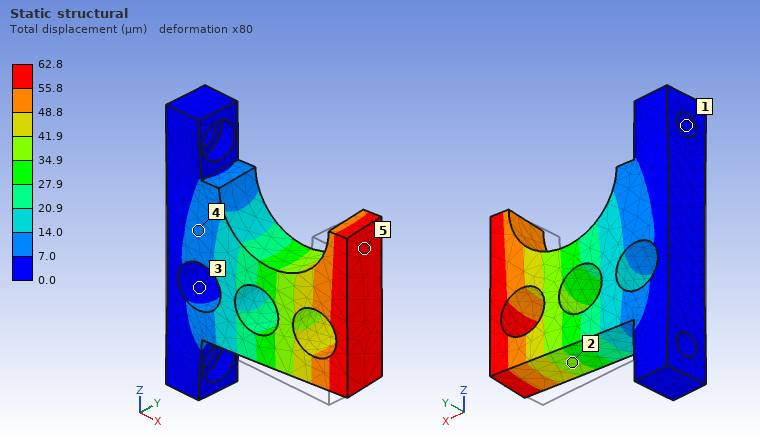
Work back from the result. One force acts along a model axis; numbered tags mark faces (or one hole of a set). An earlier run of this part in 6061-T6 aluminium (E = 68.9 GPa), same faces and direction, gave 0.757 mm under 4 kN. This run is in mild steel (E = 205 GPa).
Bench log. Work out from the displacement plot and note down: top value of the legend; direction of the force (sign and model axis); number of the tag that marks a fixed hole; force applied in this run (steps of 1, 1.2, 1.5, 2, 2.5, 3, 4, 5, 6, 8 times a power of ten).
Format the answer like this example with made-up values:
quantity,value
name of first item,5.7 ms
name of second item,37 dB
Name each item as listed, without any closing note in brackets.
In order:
quantity,value
top value of the legend,62.8 µm
direction of the force,+Y
number of the tag that marks a fixed hole,1
force applied in this run,1 kN
